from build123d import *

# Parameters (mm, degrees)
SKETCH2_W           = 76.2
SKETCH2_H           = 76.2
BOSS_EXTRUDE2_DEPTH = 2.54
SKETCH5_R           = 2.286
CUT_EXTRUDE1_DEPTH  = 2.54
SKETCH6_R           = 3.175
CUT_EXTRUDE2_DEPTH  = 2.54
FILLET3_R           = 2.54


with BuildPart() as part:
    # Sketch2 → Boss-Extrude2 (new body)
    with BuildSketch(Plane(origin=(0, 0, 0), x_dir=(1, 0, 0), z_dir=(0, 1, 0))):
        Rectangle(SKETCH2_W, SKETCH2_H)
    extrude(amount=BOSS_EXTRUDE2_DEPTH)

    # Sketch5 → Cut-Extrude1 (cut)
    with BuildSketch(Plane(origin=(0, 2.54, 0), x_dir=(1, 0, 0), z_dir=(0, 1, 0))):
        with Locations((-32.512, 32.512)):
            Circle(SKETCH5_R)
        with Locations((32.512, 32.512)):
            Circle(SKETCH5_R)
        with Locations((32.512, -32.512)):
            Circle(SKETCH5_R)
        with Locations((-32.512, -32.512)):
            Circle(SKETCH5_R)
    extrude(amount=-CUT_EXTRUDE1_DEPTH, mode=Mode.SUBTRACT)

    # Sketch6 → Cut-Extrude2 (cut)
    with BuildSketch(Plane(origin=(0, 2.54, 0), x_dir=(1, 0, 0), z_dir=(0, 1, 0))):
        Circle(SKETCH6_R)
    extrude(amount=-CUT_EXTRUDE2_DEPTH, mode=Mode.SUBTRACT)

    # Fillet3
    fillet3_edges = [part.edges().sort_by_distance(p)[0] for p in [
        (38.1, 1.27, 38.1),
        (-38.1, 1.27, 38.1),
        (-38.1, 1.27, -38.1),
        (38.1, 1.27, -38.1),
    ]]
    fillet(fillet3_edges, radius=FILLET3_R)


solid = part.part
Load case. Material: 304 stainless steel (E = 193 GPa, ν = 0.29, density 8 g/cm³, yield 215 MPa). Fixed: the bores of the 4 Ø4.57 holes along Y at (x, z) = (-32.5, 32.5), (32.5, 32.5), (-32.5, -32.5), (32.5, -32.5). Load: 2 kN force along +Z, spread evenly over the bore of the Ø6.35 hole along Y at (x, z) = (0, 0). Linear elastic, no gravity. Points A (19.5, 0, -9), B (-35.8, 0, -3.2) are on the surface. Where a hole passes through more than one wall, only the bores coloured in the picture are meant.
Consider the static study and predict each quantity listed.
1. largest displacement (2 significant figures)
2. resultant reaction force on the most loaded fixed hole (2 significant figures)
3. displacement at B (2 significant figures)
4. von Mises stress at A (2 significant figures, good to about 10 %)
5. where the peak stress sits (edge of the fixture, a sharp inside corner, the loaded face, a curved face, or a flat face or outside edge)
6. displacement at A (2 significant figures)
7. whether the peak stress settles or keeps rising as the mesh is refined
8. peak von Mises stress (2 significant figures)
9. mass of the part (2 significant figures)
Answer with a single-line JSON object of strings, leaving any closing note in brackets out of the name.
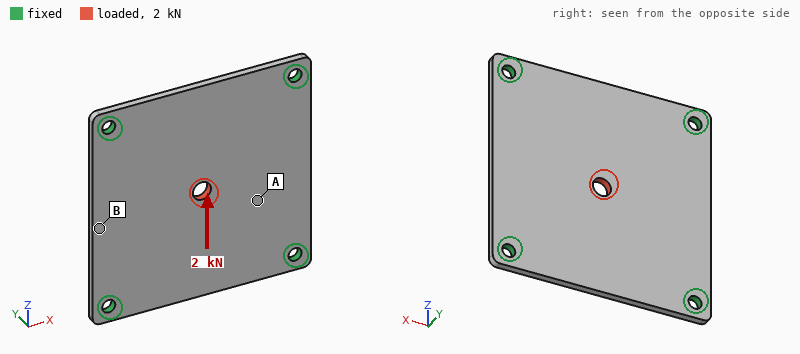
{"largest displacement": "4.4 µm", "resultant reaction force on the most loaded fixed hole": "570 N", "displacement at B": "0.96 µm", "von Mises stress at A": "10.0 MPa", "where the peak stress sits": "the loaded face", "displacement at A": "1.7 µm", "whether the peak stress settles or keeps rising as the mesh is refined": "settles", "peak von Mises stress": "70 MPa", "mass of the part": "120 g"}
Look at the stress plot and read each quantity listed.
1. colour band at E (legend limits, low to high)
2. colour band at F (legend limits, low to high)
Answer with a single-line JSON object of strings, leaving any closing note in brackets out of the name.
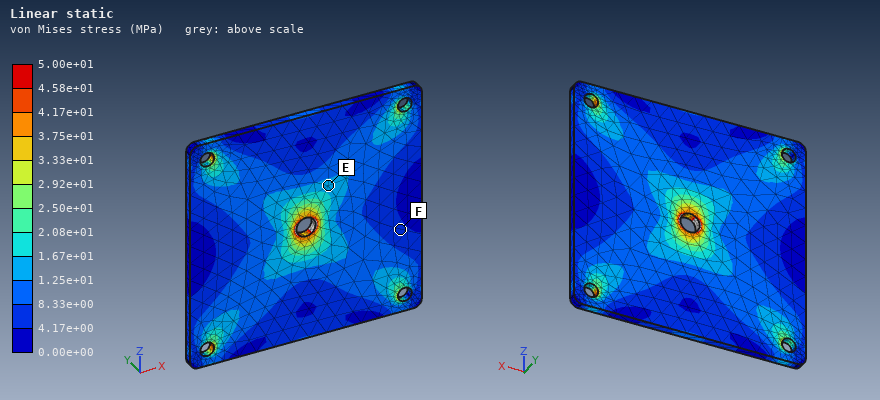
{"colour band at E": "1.25e+01 to 1.67e+01 MPa", "colour band at F": "4.17e+00 to 8.33e+00 MPa"}
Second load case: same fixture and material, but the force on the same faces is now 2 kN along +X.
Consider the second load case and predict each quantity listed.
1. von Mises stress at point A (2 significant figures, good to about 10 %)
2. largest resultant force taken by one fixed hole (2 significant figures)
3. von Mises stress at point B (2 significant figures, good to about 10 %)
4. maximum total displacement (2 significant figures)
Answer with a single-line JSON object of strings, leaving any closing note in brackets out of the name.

{"von Mises stress at point A": "9.9 MPa", "largest resultant force taken by one fixed hole": "570 N", "von Mises stress at point B": "6.7 MPa", "maximum total displacement": "4.4 µm"}
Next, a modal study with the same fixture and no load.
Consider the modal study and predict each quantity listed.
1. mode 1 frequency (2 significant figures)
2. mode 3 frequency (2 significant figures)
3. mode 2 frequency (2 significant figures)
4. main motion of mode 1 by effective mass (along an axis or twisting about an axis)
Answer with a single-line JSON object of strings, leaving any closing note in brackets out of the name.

{"mode 1 frequency": "2000 Hz", "mode 3 frequency": "3500 Hz", "mode 2 frequency": "3500 Hz", "main motion of mode 1 by effective mass": "along Y"}
